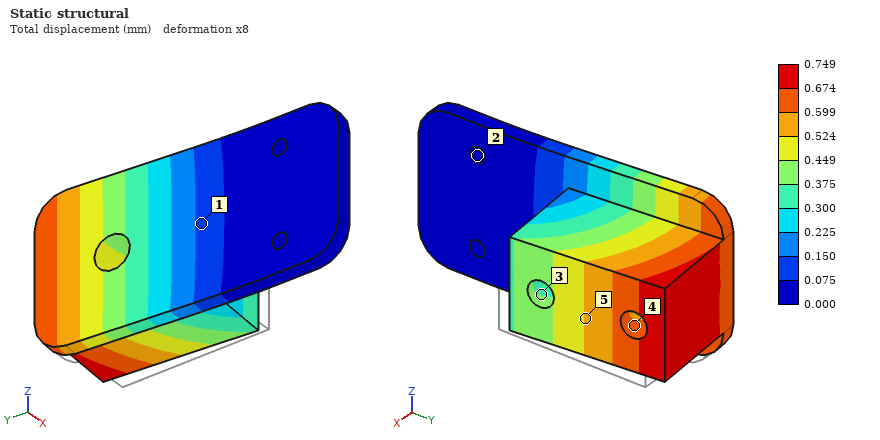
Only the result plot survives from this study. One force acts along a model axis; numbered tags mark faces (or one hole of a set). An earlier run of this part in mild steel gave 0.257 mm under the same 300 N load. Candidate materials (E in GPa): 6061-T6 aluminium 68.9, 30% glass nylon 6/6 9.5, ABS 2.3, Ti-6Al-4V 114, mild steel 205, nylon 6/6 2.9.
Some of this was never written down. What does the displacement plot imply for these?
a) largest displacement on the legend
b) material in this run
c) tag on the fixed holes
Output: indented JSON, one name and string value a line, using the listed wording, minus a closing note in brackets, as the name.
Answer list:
{
  "largest displacement on the legend": "0.749 mm",
  "material in this run": "6061-T6 aluminium",
  "tag on the fixed holes": "2"
}
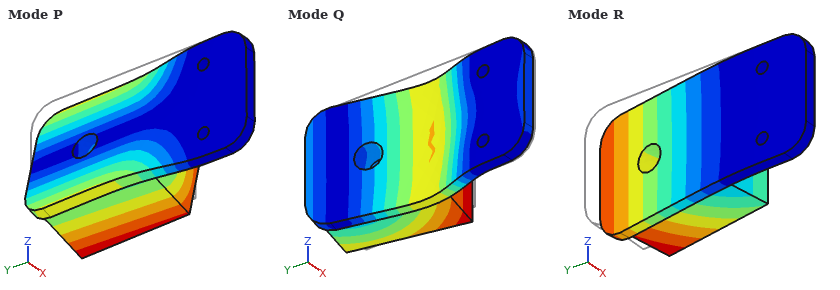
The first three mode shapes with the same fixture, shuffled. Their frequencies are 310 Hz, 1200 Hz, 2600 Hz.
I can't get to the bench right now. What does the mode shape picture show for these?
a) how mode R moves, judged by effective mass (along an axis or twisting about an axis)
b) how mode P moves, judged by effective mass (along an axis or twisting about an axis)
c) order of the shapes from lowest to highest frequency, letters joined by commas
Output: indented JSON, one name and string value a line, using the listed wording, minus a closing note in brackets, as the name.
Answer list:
{
  "how mode R moves, judged by effective mass": "along X",
  "how mode P moves, judged by effective mass": "along Z",
  "order of the shapes from lowest to highest frequency, letters joined by commas": "R, P, Q"
}
